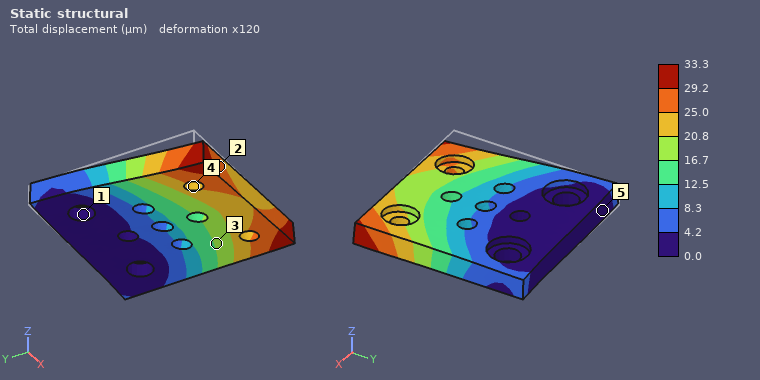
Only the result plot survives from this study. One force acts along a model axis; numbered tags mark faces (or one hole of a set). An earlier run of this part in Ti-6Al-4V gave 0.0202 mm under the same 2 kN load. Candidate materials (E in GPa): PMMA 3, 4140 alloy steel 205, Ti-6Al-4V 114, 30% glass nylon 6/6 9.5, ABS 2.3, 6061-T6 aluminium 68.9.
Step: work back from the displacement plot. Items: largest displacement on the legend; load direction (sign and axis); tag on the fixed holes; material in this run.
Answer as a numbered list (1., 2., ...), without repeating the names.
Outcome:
1. 33.3 µm
2. +X
3. 1
4. 6061-T6 aluminium
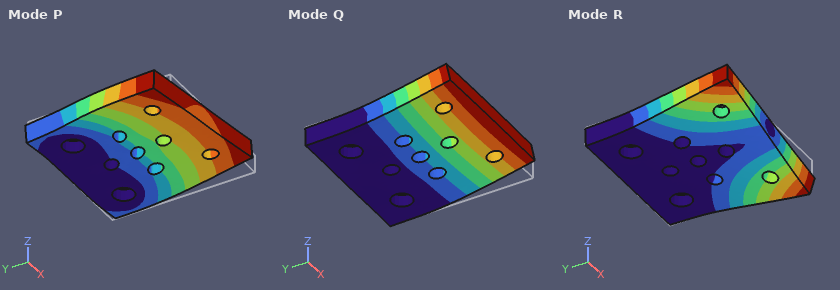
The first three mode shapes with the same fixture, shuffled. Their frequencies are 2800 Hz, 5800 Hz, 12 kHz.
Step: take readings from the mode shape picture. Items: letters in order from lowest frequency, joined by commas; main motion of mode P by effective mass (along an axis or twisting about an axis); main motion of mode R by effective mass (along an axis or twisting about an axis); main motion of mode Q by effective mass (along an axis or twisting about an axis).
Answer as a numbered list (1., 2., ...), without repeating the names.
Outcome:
1. Q, R, P
2. along X
3. twisting about Y
4. along Z
